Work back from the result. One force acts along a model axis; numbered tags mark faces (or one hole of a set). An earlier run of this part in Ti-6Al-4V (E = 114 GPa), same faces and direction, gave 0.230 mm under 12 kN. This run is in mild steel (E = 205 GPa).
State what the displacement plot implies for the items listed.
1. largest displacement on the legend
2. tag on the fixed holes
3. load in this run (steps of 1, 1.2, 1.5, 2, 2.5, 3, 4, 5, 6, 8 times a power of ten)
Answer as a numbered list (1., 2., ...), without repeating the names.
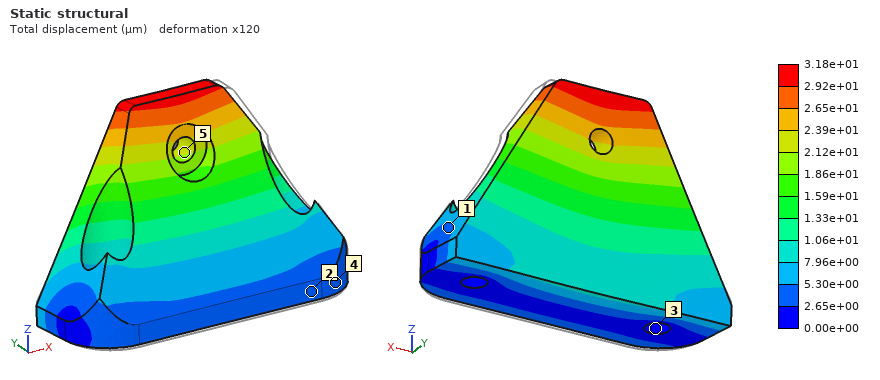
1. 3.18e+01 µm
2. 3
3. 3 kN
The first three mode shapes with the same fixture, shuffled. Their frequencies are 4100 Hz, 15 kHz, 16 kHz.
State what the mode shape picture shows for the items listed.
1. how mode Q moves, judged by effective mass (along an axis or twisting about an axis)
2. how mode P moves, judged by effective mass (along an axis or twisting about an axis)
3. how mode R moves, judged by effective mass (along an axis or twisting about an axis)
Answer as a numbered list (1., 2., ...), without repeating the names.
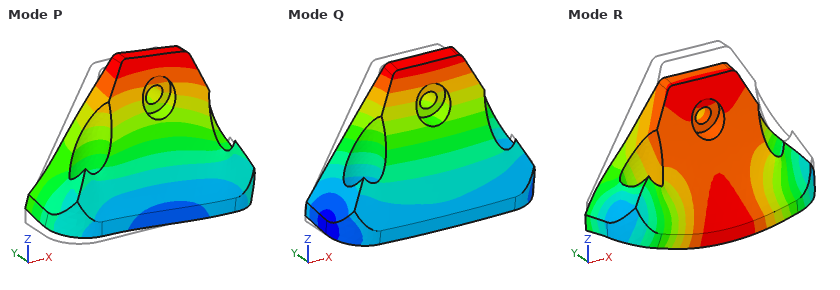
1. along Y
2. along X
3. along Z
